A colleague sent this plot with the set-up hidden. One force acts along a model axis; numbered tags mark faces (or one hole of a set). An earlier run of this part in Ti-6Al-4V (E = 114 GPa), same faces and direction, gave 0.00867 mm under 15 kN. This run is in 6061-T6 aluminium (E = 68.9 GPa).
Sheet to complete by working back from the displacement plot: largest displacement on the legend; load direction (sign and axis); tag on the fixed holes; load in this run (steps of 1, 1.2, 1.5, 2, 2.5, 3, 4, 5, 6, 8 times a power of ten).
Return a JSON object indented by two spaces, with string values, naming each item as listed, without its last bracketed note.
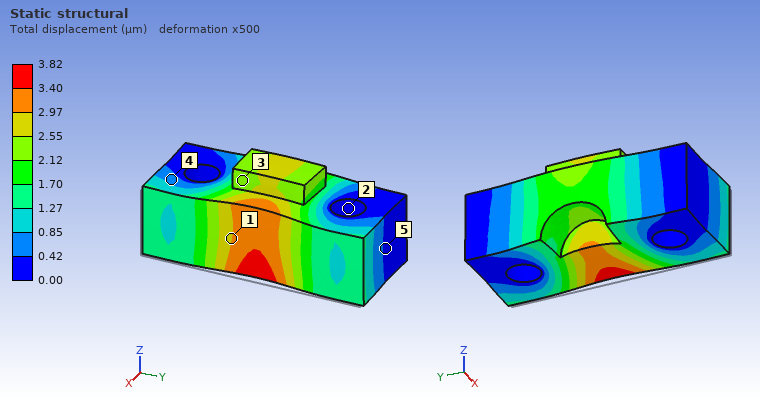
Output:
{
  "largest displacement on the legend": "3.82 µm",
  "load direction": "-X",
  "tag on the fixed holes": "2",
  "load in this run": "4 kN"
}
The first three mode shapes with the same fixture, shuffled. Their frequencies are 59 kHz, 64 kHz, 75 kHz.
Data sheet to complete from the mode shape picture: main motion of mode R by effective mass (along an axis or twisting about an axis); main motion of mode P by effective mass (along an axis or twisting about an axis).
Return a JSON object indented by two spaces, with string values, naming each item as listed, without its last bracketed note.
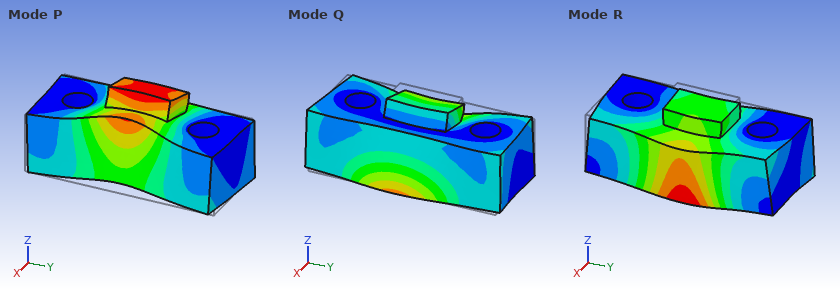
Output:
{
  "main motion of mode R by effective mass": "along Z",
  "main motion of mode P by effective mass": "along X"
}
